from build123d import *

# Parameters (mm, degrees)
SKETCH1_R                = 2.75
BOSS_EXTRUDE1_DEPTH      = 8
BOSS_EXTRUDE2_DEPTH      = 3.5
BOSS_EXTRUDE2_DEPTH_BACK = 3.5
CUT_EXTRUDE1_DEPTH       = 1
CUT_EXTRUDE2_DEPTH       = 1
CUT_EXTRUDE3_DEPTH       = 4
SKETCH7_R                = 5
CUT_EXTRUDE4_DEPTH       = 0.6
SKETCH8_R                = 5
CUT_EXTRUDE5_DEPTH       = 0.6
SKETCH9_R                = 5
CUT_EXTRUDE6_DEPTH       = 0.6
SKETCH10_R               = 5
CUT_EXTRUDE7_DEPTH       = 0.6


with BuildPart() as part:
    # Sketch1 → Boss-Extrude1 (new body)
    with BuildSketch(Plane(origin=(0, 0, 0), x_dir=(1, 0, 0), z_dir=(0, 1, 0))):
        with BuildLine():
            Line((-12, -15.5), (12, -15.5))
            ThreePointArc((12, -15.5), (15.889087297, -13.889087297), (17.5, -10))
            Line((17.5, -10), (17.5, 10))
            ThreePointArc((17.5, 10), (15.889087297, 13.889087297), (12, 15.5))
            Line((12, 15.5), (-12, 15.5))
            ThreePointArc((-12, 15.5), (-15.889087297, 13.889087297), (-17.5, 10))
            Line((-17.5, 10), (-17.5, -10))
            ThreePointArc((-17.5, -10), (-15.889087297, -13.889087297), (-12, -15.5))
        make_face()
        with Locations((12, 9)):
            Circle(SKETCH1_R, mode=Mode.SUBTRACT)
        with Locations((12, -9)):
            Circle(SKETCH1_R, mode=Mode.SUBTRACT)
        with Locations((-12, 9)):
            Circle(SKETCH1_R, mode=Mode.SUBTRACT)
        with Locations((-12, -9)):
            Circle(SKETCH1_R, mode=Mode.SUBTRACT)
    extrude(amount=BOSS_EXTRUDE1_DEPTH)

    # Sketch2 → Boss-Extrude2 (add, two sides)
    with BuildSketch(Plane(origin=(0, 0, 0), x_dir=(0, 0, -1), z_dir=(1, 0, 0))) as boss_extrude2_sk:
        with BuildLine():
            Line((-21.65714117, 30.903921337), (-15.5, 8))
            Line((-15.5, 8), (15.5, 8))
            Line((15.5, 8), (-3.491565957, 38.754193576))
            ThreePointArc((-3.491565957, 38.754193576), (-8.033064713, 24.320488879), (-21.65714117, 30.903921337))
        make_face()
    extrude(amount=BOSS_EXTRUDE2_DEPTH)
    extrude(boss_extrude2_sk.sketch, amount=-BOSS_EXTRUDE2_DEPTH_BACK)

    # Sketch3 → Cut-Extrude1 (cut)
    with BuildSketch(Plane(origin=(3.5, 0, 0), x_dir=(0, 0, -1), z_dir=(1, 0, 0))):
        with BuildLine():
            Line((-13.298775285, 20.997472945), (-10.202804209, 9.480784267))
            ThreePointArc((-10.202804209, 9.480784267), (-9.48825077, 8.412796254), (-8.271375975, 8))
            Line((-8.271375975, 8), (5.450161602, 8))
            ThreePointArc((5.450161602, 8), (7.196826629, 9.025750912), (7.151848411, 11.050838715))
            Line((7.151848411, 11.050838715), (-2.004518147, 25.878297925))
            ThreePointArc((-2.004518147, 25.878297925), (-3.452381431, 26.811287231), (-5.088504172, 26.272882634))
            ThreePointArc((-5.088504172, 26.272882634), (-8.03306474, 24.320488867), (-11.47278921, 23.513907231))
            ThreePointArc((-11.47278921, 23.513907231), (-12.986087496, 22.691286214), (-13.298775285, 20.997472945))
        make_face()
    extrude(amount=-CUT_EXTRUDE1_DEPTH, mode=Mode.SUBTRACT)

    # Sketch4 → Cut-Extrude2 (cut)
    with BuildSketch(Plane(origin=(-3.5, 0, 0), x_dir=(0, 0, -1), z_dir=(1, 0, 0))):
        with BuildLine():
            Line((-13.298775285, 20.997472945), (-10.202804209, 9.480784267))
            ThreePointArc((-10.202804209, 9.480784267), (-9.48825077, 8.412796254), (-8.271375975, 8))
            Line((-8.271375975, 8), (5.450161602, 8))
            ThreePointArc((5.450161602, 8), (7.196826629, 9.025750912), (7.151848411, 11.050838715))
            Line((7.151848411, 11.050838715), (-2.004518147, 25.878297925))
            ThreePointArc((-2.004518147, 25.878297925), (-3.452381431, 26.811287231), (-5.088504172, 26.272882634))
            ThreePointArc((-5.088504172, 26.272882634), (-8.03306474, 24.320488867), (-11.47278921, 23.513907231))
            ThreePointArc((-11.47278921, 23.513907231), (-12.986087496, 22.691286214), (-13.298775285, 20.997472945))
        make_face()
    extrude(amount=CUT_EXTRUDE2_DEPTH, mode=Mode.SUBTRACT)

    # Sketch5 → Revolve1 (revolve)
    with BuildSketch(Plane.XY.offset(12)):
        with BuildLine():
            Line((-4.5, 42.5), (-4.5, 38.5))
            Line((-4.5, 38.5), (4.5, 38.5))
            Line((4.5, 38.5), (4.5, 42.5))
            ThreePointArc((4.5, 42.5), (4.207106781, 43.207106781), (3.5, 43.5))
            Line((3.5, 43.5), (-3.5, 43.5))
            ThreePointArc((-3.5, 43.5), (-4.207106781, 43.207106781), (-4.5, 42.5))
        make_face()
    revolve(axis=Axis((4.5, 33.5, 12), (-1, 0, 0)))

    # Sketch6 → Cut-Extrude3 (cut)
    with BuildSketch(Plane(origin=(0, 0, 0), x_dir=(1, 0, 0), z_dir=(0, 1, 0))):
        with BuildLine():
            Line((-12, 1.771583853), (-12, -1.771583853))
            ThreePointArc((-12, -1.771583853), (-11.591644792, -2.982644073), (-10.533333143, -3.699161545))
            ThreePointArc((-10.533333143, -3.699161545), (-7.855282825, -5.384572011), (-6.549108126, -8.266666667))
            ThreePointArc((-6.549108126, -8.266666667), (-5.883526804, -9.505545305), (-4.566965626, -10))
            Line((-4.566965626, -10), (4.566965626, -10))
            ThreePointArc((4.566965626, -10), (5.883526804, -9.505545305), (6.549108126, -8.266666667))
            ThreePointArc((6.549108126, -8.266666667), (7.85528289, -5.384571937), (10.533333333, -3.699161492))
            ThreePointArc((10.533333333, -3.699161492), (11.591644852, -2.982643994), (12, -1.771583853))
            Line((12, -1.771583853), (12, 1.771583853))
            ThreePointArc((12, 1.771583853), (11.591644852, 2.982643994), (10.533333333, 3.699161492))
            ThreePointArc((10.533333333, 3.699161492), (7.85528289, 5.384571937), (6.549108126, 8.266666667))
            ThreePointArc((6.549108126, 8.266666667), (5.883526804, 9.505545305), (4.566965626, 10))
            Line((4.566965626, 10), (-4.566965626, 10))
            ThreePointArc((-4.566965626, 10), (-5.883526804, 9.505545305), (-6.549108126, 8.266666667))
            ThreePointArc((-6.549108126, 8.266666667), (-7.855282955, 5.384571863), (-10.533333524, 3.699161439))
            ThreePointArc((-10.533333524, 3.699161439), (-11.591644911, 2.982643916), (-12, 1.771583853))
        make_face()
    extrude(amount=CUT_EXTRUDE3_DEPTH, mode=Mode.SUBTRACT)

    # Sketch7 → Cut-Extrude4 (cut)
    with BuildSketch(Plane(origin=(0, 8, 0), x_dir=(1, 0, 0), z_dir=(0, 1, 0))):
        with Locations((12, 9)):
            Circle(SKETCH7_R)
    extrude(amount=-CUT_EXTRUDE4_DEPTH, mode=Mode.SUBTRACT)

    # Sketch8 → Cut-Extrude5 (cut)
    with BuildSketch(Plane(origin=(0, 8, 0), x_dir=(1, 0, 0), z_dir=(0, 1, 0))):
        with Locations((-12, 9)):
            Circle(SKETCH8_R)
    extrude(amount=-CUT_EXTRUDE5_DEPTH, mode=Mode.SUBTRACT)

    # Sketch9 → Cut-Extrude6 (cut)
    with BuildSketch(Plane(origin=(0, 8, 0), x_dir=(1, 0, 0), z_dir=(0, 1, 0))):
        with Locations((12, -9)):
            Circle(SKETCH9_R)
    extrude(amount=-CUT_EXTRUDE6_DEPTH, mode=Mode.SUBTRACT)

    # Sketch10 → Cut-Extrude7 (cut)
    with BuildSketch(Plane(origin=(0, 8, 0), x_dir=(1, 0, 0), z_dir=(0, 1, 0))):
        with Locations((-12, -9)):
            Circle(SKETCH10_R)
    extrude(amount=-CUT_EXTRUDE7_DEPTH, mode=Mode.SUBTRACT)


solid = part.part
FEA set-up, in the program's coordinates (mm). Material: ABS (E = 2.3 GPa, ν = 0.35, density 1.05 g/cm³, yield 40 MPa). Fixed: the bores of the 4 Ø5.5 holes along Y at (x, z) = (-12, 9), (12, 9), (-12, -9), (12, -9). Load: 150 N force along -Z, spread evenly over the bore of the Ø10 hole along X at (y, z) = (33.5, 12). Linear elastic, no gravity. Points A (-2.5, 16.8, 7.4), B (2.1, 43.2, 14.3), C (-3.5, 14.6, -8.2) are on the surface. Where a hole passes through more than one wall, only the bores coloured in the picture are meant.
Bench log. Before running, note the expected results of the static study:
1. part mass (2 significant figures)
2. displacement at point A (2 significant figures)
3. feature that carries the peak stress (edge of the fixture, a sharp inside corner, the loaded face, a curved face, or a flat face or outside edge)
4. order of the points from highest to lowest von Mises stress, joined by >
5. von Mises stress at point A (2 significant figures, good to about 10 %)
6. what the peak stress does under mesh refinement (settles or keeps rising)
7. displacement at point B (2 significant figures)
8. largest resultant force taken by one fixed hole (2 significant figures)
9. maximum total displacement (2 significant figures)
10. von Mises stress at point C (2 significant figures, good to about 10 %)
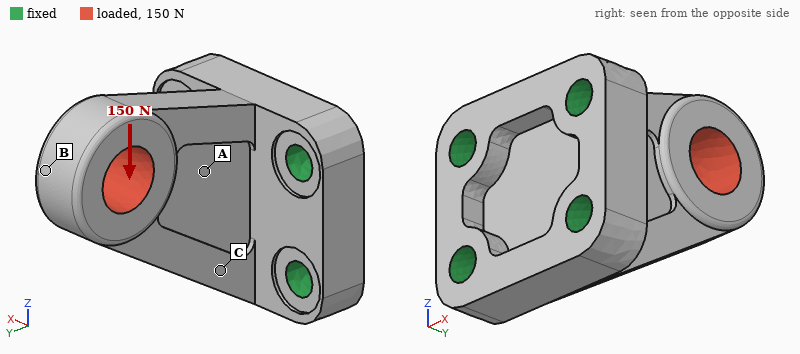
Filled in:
12 g
0.050 mm
edge of the fixture
C > A > B
2.2 MPa
keeps rising
0.20 mm
110 N
0.20 mm
3.4 MPa
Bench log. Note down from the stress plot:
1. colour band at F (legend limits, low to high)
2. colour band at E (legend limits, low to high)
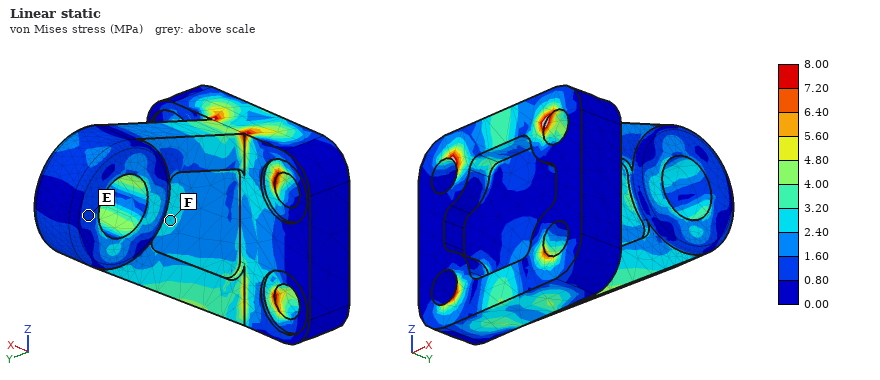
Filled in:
2.40 to 3.20 MPa
0.80 to 1.60 MPa
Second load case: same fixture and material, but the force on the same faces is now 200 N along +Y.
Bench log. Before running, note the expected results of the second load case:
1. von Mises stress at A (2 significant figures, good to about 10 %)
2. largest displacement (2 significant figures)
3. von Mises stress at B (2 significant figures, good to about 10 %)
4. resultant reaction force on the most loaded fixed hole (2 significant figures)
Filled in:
1.8 MPa
0.11 mm
1.5 MPa
110 N
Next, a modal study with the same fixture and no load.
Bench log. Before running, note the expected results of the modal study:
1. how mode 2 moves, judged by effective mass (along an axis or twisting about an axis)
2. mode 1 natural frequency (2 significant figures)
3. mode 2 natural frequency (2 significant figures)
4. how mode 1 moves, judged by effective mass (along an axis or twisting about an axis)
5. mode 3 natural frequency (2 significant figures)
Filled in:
along Z
1100 Hz
2800 Hz
along X
3500 Hz
